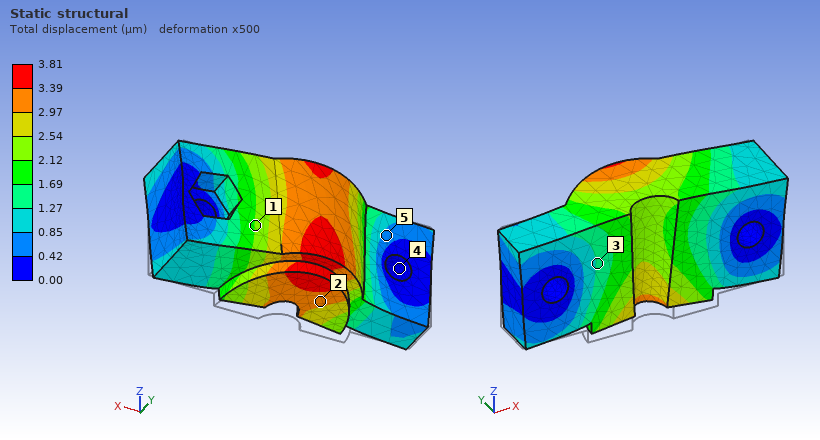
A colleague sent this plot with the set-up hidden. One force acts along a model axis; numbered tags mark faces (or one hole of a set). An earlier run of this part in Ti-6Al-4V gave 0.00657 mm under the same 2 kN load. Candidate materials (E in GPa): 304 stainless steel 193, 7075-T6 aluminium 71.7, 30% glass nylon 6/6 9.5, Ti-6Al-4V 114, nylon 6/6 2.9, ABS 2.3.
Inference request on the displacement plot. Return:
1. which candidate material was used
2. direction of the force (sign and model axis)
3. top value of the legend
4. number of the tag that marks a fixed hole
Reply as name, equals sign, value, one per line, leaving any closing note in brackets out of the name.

which candidate material was used = 304 stainless steel
direction of the force = +Z
top value of the legend = 3.81 µm
number of the tag that marks a fixed hole = 4
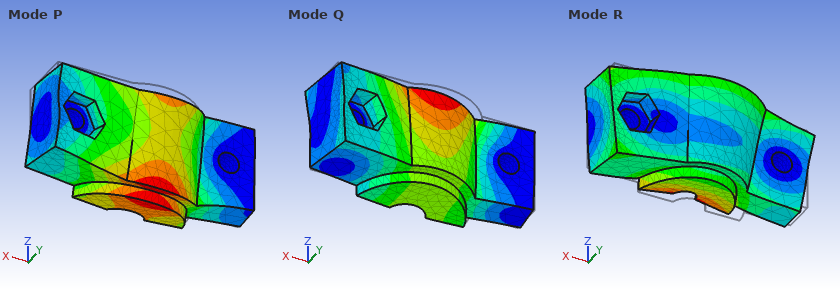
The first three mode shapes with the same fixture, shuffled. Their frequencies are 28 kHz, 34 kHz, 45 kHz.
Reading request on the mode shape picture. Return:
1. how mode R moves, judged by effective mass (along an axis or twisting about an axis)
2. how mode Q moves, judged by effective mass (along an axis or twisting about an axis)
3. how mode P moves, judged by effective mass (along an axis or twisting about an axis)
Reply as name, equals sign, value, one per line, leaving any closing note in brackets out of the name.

how mode R moves, judged by effective mass = along Z
how mode Q moves, judged by effective mass = along Y
how mode P moves, judged by effective mass = along Z
